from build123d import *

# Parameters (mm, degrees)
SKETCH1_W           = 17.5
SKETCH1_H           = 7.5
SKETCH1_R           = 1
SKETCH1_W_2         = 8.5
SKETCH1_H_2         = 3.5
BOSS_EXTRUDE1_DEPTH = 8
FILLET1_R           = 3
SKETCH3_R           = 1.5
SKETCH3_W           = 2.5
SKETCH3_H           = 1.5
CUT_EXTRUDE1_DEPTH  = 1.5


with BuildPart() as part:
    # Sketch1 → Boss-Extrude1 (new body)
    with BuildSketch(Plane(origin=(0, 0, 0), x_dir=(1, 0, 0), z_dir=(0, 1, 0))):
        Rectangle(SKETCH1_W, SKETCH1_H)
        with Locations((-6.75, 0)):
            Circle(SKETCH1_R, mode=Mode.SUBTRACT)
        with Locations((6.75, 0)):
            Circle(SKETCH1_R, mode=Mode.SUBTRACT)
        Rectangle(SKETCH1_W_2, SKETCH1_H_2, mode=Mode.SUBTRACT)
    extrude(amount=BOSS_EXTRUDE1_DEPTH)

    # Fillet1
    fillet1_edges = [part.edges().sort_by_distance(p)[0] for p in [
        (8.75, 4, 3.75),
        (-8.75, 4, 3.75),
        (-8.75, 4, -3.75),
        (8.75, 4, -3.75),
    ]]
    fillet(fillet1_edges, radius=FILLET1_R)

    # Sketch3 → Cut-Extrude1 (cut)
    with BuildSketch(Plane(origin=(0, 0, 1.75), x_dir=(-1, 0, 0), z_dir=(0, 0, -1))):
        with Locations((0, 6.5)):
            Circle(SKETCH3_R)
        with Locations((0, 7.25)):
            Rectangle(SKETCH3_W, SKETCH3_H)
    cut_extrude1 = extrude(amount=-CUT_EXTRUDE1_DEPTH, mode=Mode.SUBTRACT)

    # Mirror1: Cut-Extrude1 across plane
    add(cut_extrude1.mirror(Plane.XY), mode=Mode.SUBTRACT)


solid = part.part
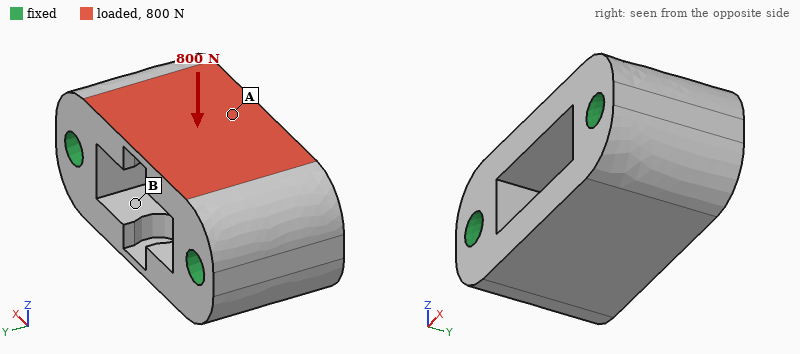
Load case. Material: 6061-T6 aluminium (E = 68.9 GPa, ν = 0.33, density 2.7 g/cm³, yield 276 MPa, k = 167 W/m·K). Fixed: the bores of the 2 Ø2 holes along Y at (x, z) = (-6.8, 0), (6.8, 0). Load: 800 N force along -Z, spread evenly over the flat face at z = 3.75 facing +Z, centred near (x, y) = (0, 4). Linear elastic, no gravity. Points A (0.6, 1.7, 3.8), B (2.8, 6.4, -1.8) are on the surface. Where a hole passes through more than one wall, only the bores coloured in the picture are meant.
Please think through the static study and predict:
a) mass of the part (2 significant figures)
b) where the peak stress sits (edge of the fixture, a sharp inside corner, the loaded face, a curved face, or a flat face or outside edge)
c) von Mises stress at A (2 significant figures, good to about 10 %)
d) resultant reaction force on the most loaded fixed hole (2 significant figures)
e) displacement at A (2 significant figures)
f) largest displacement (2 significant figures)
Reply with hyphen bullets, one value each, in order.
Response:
- 1.8 g
- the loaded face
- 68 MPa
- 450 N
- 8.6 µm
- 13 µm
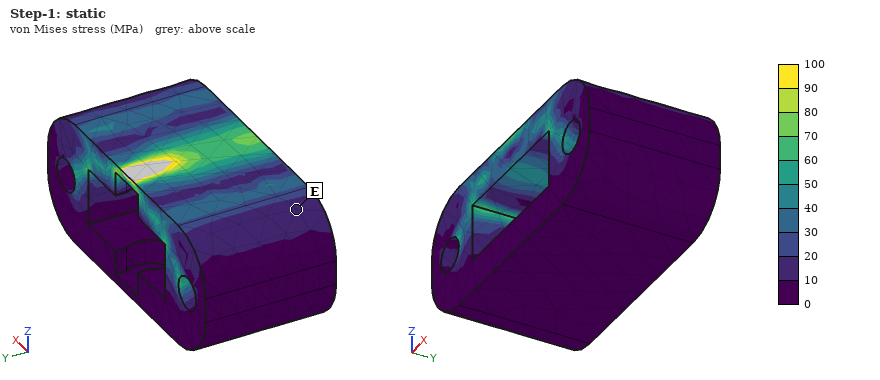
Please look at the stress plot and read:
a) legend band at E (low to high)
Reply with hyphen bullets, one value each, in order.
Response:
- 10 to 20 MPa
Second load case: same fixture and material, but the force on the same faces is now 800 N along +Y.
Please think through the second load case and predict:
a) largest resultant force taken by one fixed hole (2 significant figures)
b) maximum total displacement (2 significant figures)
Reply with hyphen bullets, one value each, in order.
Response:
- 400 N
- 10 µm
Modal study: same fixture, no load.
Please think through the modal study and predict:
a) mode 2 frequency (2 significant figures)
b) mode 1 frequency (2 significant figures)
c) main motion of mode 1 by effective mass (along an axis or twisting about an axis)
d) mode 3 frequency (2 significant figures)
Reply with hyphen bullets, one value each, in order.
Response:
- 82 kHz
- 77 kHz
- along Z
- 98 kHz
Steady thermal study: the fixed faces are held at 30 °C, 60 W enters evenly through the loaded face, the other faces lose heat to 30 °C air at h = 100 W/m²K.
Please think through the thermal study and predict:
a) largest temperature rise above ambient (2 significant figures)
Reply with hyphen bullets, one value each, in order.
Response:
- 48 K
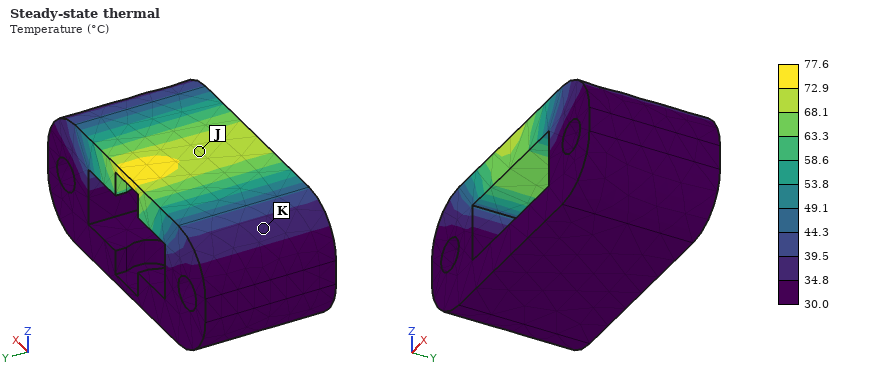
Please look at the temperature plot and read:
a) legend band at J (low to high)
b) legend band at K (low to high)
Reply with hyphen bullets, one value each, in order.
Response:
- 68.1 to 72.9 °C
- 34.8 to 39.5 °C
